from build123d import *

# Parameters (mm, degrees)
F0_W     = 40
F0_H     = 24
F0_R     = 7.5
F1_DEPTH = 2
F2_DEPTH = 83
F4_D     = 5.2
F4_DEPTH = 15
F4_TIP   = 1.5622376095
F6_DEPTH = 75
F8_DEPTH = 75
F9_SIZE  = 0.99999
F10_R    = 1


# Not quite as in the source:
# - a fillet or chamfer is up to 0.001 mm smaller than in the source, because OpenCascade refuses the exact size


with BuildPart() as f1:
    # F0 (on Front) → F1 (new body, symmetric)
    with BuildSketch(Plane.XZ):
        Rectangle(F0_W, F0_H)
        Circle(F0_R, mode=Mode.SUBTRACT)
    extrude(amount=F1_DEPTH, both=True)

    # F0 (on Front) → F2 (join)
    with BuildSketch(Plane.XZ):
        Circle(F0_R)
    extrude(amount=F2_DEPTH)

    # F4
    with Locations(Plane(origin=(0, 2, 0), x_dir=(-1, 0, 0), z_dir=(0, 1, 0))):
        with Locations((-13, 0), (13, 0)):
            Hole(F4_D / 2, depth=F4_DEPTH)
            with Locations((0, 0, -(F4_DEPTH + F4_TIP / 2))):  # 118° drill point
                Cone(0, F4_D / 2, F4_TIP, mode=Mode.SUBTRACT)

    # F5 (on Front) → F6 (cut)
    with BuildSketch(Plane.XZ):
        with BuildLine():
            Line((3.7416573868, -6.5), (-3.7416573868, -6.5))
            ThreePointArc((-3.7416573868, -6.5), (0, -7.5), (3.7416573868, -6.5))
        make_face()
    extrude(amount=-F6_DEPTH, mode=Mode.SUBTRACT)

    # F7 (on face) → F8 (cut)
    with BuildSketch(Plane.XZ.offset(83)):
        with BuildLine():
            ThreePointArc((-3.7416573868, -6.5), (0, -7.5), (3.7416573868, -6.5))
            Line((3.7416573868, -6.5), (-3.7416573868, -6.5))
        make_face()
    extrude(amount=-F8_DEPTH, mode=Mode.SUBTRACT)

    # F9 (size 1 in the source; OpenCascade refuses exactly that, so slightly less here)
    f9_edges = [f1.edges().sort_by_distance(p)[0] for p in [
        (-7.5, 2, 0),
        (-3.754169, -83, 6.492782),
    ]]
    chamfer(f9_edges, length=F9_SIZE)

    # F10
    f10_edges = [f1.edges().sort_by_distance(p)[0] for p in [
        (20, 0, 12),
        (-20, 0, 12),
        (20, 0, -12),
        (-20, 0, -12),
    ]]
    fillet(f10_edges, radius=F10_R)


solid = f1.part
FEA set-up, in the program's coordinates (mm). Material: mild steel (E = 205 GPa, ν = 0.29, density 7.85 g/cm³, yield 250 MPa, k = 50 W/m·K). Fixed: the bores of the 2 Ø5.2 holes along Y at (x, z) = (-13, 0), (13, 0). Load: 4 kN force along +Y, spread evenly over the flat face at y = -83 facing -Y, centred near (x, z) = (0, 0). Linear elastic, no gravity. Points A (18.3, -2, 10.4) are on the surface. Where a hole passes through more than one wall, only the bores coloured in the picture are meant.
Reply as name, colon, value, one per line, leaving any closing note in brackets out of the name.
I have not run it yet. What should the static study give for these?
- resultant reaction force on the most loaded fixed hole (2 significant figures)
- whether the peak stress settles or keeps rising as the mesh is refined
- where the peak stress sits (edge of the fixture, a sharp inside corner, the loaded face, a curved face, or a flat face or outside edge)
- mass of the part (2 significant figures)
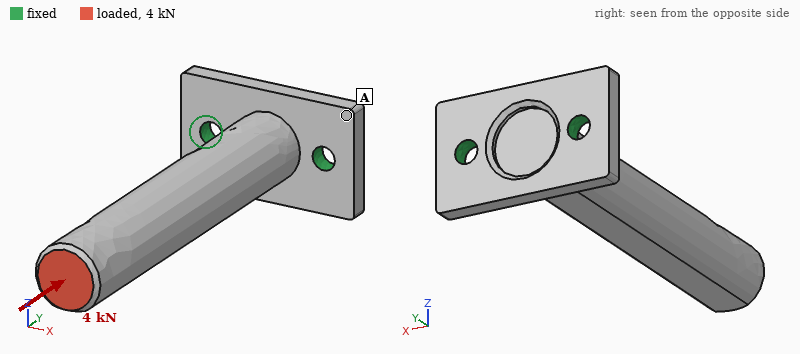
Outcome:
resultant reaction force on the most loaded fixed hole: 2.3 kN
whether the peak stress settles or keeps rising as the mesh is refined: keeps rising
where the peak stress sits: edge of the fixture
mass of the part: 140 g
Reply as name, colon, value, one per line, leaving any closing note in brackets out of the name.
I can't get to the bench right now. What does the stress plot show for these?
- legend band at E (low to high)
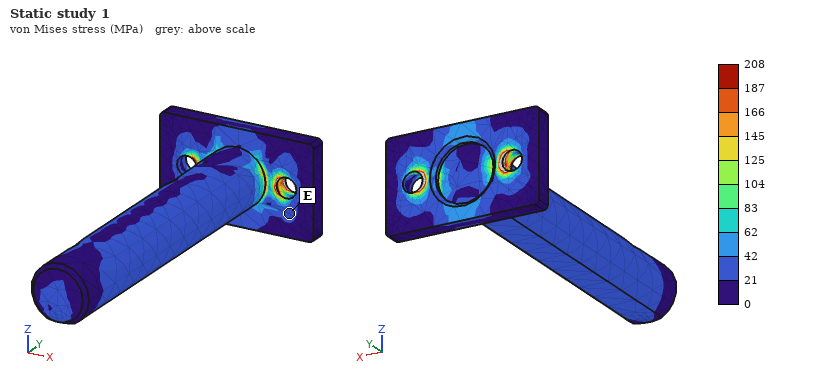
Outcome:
legend band at E: 21 to 42 MPa
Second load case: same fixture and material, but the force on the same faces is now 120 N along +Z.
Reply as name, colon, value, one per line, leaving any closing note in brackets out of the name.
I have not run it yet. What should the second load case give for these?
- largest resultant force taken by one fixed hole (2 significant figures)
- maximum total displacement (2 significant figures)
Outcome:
largest resultant force taken by one fixed hole: 61 N
maximum total displacement: 0.13 mm
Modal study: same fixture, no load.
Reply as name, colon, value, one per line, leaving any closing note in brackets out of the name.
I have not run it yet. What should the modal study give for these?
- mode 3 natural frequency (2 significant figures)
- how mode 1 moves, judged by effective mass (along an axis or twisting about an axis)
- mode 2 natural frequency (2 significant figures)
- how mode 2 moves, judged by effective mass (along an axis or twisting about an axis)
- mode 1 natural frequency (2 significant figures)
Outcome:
mode 3 natural frequency: 6700 Hz
how mode 1 moves, judged by effective mass: along Z
mode 2 natural frequency: 1300 Hz
how mode 2 moves, judged by effective mass: along X
mode 1 natural frequency: 830 Hz
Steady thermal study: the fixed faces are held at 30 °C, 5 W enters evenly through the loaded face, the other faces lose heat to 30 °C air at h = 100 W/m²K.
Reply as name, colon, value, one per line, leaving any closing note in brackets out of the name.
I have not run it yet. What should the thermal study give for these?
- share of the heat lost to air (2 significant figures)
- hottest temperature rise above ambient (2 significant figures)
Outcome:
share of the heat lost to air: 79 %
hottest temperature rise above ambient: 25 K
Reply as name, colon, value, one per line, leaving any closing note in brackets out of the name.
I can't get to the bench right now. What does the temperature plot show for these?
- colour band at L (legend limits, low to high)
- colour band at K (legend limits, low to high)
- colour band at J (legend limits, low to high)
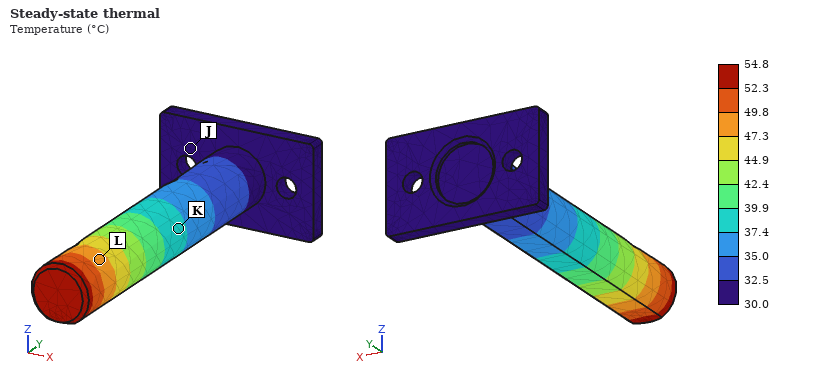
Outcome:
colour band at L: 47.3 to 49.8 °C
colour band at K: 37.4 to 39.9 °C
colour band at J: 30.0 to 32.5 °C
